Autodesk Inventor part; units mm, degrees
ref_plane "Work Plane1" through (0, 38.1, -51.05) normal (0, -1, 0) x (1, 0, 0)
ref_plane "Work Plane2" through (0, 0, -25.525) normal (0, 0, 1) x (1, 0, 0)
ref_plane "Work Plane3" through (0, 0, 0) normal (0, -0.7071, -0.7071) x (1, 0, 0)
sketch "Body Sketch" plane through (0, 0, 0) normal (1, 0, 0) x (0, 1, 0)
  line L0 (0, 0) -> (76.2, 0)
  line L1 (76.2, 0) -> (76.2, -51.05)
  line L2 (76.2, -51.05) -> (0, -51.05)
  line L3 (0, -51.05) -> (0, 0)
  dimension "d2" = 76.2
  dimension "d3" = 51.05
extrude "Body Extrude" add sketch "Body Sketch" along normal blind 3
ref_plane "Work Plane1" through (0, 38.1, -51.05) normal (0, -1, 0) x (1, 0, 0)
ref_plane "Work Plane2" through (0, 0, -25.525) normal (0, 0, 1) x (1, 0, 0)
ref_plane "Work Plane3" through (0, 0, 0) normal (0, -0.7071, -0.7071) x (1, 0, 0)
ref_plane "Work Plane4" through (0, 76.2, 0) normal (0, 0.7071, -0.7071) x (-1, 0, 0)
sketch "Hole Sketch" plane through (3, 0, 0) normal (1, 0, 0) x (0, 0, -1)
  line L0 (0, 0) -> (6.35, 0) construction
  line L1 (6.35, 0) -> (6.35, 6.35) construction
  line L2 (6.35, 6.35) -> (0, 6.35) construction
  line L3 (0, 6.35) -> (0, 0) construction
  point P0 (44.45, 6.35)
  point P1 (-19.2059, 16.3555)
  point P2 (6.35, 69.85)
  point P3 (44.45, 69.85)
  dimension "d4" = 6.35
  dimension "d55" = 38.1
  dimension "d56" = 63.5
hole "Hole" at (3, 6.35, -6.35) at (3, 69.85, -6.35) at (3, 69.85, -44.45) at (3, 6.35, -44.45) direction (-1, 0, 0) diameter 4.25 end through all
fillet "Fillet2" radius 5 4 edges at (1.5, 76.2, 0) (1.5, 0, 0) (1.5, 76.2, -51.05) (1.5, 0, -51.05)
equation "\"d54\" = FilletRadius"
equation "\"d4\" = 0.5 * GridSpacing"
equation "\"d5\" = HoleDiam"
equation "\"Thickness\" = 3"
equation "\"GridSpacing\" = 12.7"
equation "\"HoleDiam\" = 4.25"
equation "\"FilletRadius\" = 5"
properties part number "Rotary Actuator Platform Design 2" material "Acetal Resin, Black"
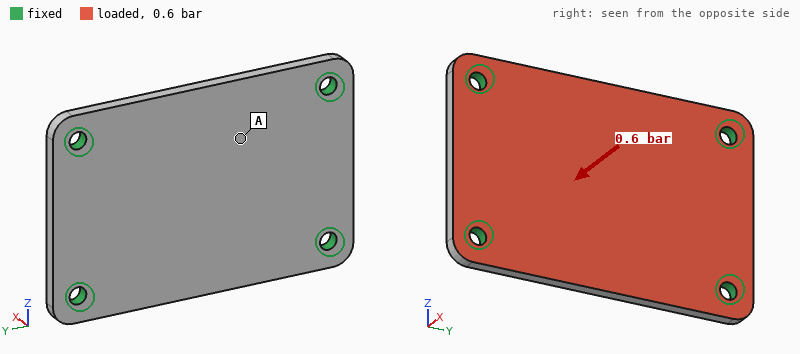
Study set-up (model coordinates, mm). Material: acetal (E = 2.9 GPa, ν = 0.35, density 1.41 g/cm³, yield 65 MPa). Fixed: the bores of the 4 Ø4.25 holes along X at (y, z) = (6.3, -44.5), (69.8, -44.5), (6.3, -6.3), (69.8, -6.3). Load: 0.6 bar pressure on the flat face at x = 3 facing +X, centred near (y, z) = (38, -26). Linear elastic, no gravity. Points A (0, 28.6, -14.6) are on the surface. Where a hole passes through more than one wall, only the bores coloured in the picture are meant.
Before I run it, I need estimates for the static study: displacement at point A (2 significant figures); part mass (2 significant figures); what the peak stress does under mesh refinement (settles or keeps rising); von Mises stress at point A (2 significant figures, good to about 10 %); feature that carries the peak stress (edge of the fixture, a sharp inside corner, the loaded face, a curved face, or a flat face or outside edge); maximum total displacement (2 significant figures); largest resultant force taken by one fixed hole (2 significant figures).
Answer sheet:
0.38 mm
16 g
keeps rising
4.9 MPa
edge of the fixture
0.46 mm
58 N
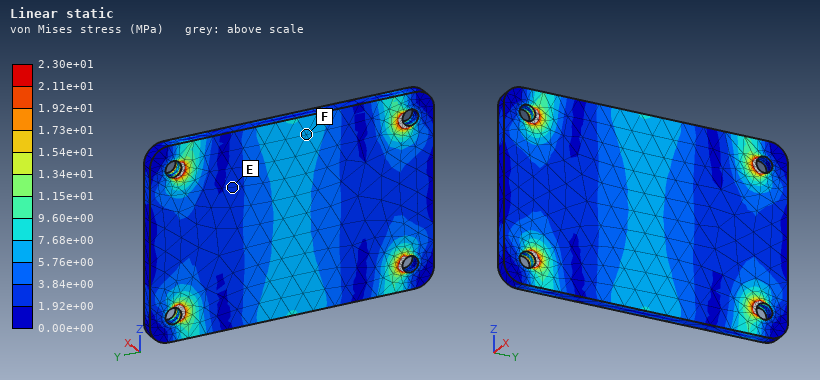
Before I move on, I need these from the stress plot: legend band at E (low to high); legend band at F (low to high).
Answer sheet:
1.92e+00 to 3.84e+00 MPa
5.76e+00 to 7.68e+00 MPa
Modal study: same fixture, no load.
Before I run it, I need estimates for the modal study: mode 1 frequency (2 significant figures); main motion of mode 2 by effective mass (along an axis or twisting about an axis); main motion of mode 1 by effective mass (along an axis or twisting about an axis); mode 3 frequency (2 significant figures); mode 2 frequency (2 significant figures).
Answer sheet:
1000 Hz
twisting about Y
along X
2500 Hz
1500 Hz
